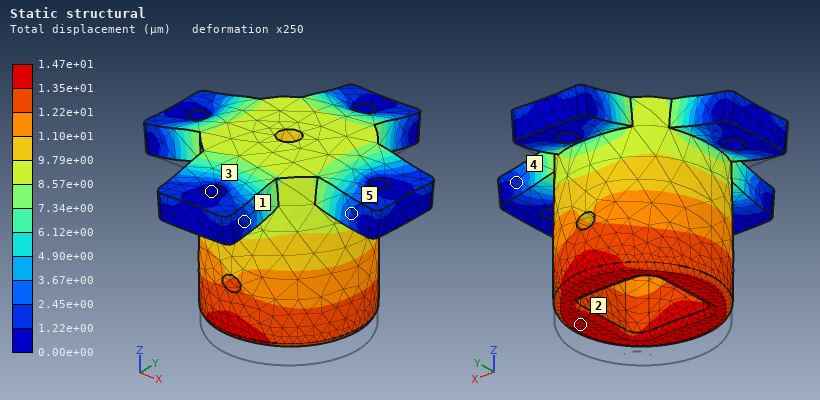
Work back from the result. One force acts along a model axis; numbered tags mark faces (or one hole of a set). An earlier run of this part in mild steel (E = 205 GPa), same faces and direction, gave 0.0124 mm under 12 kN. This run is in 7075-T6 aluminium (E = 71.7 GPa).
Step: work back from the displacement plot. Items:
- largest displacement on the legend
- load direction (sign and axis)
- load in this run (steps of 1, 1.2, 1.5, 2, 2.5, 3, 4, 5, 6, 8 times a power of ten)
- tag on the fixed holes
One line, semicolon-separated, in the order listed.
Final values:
1.47e+01 µm; +Z; 5 kN; 3
